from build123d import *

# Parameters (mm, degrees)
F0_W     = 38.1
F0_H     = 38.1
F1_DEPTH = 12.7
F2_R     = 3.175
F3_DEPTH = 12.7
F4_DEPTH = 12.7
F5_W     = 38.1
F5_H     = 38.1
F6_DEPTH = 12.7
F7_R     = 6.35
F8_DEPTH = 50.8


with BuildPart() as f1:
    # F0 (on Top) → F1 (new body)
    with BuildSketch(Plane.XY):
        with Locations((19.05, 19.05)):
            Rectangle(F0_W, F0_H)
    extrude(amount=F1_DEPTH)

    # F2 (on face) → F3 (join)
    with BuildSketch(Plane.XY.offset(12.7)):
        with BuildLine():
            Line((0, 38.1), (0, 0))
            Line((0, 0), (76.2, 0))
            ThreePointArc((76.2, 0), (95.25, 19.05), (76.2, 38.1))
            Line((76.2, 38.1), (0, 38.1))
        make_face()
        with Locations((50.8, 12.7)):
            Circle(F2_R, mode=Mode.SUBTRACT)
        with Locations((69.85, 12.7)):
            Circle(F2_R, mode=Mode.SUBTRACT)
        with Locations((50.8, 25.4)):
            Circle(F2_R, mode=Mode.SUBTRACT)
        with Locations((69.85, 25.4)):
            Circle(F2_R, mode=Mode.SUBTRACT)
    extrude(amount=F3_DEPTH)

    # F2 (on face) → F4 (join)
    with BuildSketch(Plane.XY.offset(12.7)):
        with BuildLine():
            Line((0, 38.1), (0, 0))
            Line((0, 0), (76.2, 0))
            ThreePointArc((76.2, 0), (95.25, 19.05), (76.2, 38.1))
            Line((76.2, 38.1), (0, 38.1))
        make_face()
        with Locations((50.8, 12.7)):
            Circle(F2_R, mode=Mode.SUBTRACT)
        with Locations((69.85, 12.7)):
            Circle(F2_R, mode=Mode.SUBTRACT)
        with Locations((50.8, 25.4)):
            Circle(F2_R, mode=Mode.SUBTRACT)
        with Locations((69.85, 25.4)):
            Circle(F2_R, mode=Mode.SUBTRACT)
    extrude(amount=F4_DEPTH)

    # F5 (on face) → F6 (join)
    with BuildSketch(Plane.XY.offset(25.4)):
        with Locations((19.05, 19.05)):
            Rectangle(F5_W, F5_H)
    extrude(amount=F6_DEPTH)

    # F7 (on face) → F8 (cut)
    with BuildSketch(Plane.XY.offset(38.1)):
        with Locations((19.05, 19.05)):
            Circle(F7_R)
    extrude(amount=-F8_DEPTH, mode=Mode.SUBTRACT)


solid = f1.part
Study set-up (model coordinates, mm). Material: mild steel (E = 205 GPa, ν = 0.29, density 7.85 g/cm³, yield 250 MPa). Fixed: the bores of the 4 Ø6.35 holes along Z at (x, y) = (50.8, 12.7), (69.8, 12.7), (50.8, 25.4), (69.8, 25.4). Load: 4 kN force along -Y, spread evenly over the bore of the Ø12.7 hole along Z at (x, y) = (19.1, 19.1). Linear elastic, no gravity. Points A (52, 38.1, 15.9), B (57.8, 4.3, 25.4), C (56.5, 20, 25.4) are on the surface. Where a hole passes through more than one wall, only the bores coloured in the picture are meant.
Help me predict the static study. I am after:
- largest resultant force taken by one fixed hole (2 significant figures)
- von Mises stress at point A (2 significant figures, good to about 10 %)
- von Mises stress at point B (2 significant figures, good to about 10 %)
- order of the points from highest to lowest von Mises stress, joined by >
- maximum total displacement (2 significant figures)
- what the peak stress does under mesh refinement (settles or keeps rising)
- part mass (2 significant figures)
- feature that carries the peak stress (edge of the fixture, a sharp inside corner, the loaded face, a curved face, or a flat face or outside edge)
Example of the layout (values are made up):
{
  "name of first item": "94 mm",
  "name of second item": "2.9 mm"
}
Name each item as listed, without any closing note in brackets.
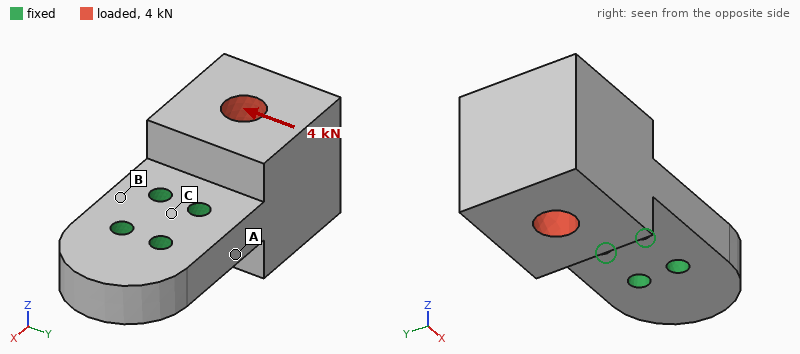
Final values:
{
  "largest resultant force taken by one fixed hole": "5.1 kN",
  "von Mises stress at point A": "30 MPa",
  "von Mises stress at point B": "16 MPa",
  "order of the points from highest to lowest von Mises stress, joined by >": "A > B > C",
  "maximum total displacement": "13 µm",
  "what the peak stress does under mesh refinement": "keeps rising",
  "part mass": "590 g",
  "feature that carries the peak stress": "edge of the fixture"
}
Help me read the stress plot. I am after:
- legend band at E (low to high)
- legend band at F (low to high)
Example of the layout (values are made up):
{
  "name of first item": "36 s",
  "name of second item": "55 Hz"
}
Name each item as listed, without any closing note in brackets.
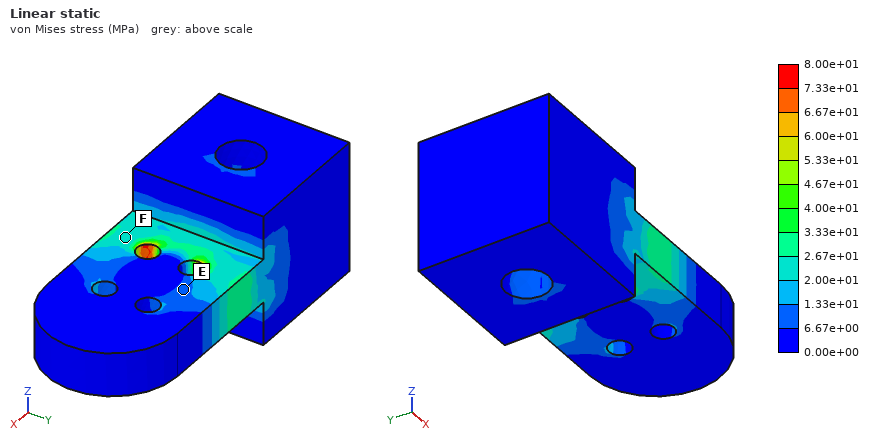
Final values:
{
  "legend band at E": "6.67e+00 to 1.33e+01 MPa",
  "legend band at F": "2.00e+01 to 2.67e+01 MPa"
}
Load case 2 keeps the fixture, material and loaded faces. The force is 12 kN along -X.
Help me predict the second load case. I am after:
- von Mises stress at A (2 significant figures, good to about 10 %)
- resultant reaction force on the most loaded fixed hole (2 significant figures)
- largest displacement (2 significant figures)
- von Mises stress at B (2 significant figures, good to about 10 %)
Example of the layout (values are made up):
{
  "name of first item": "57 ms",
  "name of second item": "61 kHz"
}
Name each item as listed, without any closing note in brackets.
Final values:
{
  "von Mises stress at A": "14 MPa",
  "resultant reaction force on the most loaded fixed hole": "5.4 kN",
  "largest displacement": "4.0 µm",
  "von Mises stress at B": "9.0 MPa"
}
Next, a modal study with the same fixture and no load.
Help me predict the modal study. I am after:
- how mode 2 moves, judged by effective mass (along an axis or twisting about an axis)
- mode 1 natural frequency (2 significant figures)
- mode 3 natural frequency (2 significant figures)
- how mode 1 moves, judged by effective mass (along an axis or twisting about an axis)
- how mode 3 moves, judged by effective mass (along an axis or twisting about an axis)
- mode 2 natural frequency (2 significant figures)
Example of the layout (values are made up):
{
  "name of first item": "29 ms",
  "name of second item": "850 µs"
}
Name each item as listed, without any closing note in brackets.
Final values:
{
  "how mode 2 moves, judged by effective mass": "along Y",
  "mode 1 natural frequency": "2500 Hz",
  "mode 3 natural frequency": "6600 Hz",
  "how mode 1 moves, judged by effective mass": "along Z",
  "how mode 3 moves, judged by effective mass": "twisting about X",
  "mode 2 natural frequency": "5100 Hz"
}
